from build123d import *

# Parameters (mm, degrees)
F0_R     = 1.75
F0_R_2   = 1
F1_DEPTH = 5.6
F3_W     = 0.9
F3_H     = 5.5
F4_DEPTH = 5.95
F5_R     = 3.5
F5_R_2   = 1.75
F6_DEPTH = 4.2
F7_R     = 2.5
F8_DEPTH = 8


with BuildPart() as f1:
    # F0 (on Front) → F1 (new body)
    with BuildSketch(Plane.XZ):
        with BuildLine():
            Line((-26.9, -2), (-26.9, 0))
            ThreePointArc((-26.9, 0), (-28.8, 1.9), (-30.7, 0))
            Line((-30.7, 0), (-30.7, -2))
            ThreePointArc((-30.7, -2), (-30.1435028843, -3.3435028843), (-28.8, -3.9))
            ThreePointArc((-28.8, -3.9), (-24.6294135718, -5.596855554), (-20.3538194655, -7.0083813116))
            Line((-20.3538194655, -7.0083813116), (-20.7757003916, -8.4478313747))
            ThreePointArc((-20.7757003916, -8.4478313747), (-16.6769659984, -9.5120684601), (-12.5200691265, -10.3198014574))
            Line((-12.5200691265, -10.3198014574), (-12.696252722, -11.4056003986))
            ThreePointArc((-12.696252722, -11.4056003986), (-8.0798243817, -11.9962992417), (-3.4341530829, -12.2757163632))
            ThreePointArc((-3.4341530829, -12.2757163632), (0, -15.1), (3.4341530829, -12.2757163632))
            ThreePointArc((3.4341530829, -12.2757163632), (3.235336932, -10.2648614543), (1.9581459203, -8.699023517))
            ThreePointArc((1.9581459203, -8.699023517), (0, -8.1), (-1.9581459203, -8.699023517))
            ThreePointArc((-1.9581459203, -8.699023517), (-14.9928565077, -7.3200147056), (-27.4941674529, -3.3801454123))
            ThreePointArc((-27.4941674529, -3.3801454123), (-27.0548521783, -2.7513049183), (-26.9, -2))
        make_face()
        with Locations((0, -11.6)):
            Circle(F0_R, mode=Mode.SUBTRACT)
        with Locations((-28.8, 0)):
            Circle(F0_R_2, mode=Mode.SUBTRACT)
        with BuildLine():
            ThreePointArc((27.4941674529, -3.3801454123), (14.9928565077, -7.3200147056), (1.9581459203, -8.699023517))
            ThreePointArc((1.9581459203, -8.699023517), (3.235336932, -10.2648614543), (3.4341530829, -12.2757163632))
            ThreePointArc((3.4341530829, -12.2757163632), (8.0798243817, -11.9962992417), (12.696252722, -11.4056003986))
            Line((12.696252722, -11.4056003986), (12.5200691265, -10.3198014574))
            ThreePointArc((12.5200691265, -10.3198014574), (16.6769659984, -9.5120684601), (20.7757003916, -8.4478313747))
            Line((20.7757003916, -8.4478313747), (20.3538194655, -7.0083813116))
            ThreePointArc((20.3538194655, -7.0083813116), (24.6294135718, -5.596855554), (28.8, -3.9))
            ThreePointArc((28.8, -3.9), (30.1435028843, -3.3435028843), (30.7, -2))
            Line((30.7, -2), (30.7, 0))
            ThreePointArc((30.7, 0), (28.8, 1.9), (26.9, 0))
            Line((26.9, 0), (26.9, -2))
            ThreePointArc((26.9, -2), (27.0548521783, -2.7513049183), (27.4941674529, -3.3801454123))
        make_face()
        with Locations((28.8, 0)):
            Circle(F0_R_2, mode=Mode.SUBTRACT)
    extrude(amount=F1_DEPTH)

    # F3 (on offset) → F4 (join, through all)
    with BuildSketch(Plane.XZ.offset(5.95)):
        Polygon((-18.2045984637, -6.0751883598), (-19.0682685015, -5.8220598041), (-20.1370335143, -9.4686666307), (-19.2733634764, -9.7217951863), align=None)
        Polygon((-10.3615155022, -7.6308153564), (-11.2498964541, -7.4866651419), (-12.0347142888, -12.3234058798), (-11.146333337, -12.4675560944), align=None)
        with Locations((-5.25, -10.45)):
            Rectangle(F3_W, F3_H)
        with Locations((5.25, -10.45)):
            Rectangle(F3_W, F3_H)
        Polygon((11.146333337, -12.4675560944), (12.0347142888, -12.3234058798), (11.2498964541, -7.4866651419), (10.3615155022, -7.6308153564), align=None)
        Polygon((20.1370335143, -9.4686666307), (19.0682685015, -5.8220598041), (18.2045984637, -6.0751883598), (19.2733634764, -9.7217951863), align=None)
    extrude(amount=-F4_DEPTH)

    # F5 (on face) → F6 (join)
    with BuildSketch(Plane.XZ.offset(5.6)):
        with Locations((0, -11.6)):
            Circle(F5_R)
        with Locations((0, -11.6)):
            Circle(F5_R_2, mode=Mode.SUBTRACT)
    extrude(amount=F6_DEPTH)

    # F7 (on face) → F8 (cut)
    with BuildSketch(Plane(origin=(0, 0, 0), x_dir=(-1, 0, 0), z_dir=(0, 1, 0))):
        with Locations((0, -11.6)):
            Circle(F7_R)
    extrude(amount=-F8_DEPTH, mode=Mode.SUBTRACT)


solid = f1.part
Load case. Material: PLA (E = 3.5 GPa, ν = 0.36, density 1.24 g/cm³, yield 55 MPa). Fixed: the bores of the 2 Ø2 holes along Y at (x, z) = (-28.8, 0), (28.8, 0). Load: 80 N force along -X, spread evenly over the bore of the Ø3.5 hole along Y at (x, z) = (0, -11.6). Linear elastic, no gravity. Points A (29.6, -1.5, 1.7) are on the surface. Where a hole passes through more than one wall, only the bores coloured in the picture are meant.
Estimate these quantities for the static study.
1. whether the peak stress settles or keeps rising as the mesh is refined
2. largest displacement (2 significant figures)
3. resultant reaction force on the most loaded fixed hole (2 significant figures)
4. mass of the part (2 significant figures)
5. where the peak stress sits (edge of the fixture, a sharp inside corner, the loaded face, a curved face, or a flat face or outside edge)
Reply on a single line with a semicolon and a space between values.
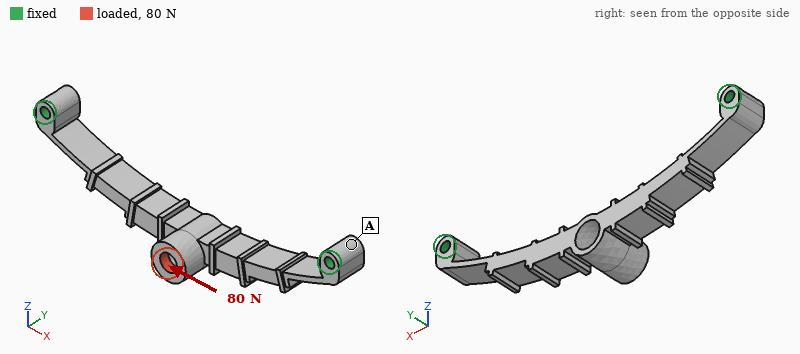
keeps rising; 0.24 mm; 43 N; 1.4 g; a sharp inside corner
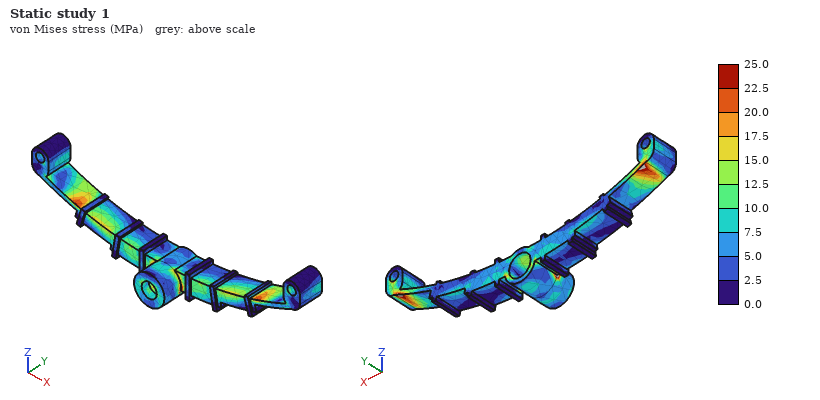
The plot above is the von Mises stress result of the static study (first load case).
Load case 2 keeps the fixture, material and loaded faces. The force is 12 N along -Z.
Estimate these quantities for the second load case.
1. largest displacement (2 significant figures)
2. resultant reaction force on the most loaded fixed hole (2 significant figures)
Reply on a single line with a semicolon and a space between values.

0.74 mm; 17 N
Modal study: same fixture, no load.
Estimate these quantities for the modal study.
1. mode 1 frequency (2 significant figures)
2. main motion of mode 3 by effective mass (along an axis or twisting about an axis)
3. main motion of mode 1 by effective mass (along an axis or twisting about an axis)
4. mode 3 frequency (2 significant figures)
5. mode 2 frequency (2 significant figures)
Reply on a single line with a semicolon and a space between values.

1000 Hz; along Z; along Y; 2100 Hz; 1900 Hz
